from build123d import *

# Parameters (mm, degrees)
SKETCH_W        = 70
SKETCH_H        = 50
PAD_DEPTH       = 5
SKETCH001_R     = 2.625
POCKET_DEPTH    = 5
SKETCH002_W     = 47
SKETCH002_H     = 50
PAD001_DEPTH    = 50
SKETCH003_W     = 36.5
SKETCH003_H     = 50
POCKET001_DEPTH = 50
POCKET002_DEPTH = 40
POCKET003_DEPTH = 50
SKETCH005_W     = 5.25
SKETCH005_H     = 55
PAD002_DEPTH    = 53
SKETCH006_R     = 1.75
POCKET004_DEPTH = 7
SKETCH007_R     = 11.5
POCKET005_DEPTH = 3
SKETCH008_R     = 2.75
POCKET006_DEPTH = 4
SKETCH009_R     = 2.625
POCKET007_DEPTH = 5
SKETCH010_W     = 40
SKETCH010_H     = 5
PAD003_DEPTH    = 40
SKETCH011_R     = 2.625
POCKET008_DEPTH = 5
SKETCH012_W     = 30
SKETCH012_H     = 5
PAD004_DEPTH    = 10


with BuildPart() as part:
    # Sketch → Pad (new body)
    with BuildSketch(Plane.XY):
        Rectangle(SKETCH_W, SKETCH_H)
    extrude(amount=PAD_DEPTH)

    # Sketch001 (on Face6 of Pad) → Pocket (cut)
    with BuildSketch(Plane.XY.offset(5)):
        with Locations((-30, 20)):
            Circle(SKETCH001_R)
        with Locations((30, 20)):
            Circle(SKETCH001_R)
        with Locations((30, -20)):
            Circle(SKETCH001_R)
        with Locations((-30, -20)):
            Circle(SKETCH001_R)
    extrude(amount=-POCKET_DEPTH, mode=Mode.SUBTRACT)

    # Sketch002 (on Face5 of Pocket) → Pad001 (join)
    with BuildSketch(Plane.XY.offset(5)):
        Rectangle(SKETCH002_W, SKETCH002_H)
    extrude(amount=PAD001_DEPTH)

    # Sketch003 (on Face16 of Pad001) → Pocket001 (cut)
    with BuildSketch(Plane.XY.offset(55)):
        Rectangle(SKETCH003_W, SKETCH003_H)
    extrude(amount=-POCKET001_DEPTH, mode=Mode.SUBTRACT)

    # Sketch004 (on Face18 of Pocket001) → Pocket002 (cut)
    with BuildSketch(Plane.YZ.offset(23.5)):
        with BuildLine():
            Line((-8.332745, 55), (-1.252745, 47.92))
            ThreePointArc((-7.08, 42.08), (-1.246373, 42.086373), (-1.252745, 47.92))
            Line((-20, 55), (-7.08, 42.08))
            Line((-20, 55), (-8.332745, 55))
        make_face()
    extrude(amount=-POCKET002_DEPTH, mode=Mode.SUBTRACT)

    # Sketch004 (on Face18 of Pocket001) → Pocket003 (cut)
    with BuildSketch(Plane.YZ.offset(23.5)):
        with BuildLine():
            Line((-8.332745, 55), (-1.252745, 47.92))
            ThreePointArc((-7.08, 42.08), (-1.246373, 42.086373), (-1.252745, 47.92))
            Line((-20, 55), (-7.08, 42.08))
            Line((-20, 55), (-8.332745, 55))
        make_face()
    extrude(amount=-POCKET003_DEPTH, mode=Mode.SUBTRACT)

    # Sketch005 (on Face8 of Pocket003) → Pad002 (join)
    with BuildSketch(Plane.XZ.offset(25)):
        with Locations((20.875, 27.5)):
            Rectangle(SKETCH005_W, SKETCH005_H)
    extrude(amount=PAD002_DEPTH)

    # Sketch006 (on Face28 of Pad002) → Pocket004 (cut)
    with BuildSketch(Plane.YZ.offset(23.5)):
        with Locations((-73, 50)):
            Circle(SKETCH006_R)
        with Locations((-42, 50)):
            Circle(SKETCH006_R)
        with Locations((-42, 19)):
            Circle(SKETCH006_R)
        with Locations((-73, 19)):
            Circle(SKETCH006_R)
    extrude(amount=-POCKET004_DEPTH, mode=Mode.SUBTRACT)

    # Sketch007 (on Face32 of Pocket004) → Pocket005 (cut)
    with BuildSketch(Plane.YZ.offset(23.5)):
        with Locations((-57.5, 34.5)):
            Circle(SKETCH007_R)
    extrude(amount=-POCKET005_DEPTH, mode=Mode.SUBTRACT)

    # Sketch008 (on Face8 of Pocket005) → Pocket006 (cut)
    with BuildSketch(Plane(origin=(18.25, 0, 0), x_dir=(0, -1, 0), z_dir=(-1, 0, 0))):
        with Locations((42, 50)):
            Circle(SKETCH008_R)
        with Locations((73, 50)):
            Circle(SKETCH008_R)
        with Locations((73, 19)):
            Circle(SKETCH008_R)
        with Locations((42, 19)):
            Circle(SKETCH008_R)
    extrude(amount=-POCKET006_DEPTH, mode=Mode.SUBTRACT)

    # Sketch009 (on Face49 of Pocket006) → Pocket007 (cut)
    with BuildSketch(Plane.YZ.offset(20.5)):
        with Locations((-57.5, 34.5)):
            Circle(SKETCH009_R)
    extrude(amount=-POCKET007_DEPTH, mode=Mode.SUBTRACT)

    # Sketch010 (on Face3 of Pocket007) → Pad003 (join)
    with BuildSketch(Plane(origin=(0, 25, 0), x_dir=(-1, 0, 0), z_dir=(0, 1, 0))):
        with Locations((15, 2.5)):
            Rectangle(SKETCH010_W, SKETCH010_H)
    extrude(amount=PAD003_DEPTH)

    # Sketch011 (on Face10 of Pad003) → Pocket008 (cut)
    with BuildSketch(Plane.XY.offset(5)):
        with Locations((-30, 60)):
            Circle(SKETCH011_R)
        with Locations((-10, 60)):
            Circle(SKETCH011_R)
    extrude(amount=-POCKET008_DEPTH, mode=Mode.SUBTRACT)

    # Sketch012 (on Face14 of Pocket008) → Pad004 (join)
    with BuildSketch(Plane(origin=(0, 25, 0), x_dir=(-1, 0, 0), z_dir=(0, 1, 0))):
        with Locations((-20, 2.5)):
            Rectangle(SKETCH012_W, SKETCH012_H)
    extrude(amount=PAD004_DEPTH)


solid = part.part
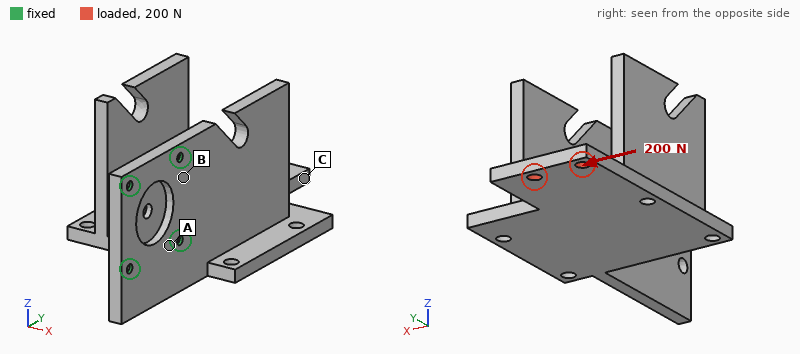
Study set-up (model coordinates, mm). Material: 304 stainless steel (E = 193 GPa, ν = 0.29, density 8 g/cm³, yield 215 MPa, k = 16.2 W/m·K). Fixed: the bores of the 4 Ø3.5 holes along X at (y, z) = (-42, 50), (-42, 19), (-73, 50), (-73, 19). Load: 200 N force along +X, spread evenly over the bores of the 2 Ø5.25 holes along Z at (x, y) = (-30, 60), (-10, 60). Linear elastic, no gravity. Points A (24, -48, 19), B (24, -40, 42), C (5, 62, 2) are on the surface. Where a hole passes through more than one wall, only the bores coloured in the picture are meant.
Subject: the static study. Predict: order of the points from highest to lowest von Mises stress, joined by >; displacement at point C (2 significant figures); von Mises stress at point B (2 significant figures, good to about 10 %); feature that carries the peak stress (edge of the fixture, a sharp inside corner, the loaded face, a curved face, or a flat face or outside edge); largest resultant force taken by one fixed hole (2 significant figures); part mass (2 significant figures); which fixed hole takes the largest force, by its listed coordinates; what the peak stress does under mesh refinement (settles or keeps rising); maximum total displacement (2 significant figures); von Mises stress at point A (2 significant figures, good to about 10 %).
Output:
B > A > C
0.58 mm
55 MPa
edge of the fixture
1.5 kN
520 g
(-42, 19)
keeps rising
0.69 mm
37 MPa
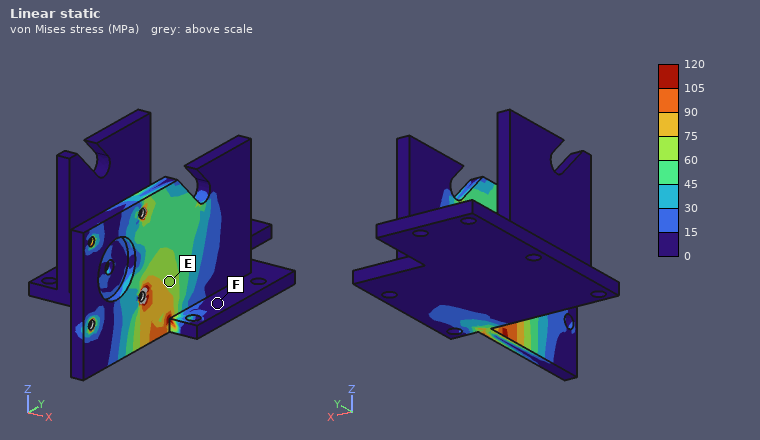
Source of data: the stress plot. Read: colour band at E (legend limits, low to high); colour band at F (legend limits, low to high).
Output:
60 to 75 MPa
0 to 15 MPa
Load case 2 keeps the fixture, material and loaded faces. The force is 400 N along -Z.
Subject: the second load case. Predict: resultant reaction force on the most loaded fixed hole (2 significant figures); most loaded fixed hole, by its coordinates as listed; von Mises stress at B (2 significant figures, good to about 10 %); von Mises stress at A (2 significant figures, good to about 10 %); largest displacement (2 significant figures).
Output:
1.5 kN
(-42, 50)
22 MPa
25 MPa
0.72 mm
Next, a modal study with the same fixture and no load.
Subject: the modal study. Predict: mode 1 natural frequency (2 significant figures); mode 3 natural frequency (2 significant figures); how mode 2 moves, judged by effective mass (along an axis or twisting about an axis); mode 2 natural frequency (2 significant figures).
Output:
250 Hz
950 Hz
along Z
380 Hz
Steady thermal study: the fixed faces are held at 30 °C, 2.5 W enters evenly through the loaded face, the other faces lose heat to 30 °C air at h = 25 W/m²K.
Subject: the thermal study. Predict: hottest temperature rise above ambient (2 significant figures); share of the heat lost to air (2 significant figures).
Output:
30 K
97 %
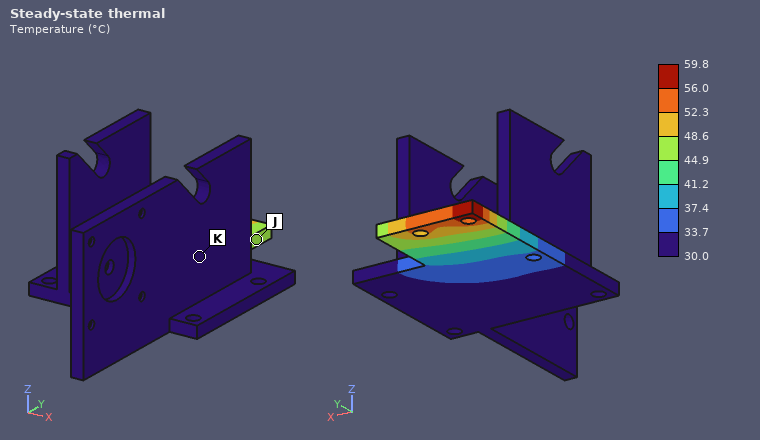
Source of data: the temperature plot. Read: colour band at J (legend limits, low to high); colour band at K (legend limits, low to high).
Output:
44.9 to 48.6 °C
30.0 to 33.7 °C
